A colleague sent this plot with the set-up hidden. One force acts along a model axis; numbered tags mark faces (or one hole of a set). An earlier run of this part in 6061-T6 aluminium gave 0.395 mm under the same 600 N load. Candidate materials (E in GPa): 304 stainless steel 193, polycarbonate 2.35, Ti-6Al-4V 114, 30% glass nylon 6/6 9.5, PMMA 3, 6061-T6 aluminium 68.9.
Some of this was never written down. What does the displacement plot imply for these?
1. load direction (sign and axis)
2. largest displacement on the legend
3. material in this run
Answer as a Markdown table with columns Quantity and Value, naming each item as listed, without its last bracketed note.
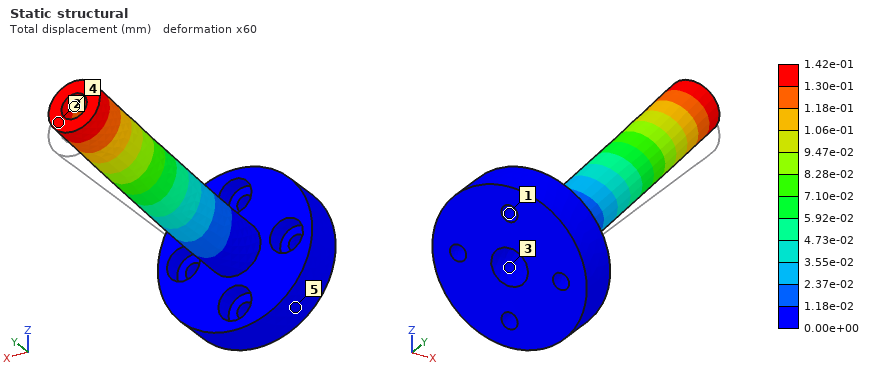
| Quantity | Value |
|---|---|
| load direction | +Z |
| largest displacement on the legend | 1.42e-01 mm |
| material in this run | 304 stainless steel |
